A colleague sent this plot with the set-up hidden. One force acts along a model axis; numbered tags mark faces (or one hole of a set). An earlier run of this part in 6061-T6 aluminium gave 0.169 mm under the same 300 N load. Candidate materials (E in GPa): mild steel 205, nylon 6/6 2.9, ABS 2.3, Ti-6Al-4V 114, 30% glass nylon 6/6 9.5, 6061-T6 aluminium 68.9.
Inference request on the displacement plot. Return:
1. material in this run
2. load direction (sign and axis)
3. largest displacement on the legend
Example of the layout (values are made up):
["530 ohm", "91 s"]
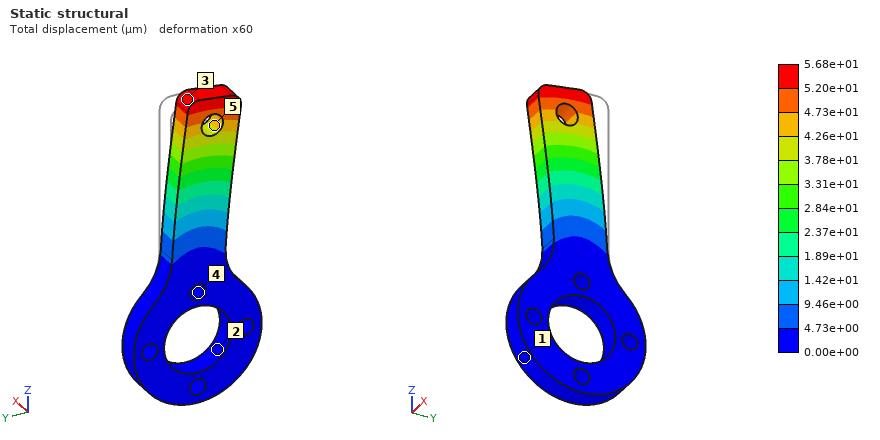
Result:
["mild steel", "-Y", "5.68e+01 µm"]
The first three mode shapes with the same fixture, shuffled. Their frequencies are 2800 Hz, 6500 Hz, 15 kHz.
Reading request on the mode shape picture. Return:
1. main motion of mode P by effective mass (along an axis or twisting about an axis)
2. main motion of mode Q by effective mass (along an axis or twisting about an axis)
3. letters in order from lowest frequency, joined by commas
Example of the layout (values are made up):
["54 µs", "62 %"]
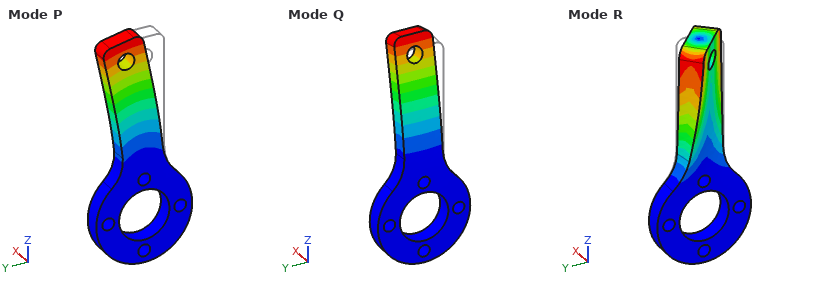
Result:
["along Y", "along X", "Q, P, R"]
